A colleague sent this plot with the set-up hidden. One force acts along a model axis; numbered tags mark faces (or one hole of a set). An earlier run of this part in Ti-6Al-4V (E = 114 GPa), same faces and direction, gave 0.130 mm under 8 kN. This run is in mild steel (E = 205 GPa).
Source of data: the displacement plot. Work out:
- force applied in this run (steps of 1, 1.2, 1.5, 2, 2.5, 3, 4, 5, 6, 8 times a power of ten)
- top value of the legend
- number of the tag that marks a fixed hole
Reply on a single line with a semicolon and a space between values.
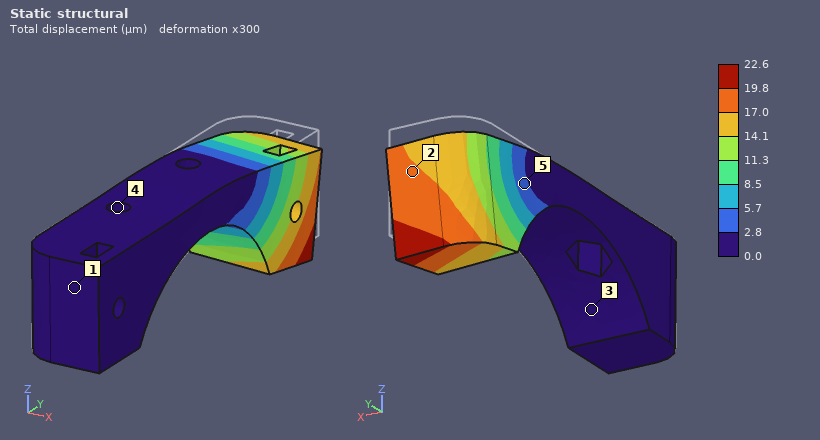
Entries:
2.5 kN; 22.6 µm; 4
